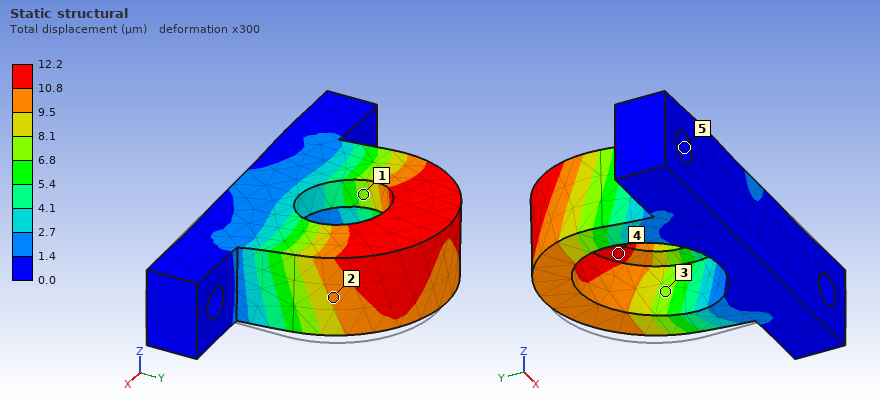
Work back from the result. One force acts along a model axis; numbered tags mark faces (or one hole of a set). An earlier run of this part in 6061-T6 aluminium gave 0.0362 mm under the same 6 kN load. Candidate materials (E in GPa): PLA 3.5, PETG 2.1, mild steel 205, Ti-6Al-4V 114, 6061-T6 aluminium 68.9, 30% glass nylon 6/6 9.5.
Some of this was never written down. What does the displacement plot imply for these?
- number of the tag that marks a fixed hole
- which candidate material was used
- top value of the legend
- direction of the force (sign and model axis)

5
mild steel
12.2 µm
-X
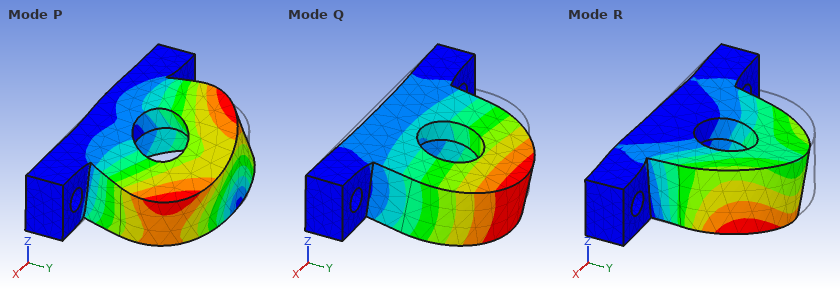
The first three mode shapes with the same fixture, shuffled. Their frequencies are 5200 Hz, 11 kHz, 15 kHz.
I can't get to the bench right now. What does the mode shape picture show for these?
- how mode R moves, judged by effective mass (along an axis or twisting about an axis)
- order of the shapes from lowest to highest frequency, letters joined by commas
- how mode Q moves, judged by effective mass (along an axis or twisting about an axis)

along X
Q, R, P
along Z
